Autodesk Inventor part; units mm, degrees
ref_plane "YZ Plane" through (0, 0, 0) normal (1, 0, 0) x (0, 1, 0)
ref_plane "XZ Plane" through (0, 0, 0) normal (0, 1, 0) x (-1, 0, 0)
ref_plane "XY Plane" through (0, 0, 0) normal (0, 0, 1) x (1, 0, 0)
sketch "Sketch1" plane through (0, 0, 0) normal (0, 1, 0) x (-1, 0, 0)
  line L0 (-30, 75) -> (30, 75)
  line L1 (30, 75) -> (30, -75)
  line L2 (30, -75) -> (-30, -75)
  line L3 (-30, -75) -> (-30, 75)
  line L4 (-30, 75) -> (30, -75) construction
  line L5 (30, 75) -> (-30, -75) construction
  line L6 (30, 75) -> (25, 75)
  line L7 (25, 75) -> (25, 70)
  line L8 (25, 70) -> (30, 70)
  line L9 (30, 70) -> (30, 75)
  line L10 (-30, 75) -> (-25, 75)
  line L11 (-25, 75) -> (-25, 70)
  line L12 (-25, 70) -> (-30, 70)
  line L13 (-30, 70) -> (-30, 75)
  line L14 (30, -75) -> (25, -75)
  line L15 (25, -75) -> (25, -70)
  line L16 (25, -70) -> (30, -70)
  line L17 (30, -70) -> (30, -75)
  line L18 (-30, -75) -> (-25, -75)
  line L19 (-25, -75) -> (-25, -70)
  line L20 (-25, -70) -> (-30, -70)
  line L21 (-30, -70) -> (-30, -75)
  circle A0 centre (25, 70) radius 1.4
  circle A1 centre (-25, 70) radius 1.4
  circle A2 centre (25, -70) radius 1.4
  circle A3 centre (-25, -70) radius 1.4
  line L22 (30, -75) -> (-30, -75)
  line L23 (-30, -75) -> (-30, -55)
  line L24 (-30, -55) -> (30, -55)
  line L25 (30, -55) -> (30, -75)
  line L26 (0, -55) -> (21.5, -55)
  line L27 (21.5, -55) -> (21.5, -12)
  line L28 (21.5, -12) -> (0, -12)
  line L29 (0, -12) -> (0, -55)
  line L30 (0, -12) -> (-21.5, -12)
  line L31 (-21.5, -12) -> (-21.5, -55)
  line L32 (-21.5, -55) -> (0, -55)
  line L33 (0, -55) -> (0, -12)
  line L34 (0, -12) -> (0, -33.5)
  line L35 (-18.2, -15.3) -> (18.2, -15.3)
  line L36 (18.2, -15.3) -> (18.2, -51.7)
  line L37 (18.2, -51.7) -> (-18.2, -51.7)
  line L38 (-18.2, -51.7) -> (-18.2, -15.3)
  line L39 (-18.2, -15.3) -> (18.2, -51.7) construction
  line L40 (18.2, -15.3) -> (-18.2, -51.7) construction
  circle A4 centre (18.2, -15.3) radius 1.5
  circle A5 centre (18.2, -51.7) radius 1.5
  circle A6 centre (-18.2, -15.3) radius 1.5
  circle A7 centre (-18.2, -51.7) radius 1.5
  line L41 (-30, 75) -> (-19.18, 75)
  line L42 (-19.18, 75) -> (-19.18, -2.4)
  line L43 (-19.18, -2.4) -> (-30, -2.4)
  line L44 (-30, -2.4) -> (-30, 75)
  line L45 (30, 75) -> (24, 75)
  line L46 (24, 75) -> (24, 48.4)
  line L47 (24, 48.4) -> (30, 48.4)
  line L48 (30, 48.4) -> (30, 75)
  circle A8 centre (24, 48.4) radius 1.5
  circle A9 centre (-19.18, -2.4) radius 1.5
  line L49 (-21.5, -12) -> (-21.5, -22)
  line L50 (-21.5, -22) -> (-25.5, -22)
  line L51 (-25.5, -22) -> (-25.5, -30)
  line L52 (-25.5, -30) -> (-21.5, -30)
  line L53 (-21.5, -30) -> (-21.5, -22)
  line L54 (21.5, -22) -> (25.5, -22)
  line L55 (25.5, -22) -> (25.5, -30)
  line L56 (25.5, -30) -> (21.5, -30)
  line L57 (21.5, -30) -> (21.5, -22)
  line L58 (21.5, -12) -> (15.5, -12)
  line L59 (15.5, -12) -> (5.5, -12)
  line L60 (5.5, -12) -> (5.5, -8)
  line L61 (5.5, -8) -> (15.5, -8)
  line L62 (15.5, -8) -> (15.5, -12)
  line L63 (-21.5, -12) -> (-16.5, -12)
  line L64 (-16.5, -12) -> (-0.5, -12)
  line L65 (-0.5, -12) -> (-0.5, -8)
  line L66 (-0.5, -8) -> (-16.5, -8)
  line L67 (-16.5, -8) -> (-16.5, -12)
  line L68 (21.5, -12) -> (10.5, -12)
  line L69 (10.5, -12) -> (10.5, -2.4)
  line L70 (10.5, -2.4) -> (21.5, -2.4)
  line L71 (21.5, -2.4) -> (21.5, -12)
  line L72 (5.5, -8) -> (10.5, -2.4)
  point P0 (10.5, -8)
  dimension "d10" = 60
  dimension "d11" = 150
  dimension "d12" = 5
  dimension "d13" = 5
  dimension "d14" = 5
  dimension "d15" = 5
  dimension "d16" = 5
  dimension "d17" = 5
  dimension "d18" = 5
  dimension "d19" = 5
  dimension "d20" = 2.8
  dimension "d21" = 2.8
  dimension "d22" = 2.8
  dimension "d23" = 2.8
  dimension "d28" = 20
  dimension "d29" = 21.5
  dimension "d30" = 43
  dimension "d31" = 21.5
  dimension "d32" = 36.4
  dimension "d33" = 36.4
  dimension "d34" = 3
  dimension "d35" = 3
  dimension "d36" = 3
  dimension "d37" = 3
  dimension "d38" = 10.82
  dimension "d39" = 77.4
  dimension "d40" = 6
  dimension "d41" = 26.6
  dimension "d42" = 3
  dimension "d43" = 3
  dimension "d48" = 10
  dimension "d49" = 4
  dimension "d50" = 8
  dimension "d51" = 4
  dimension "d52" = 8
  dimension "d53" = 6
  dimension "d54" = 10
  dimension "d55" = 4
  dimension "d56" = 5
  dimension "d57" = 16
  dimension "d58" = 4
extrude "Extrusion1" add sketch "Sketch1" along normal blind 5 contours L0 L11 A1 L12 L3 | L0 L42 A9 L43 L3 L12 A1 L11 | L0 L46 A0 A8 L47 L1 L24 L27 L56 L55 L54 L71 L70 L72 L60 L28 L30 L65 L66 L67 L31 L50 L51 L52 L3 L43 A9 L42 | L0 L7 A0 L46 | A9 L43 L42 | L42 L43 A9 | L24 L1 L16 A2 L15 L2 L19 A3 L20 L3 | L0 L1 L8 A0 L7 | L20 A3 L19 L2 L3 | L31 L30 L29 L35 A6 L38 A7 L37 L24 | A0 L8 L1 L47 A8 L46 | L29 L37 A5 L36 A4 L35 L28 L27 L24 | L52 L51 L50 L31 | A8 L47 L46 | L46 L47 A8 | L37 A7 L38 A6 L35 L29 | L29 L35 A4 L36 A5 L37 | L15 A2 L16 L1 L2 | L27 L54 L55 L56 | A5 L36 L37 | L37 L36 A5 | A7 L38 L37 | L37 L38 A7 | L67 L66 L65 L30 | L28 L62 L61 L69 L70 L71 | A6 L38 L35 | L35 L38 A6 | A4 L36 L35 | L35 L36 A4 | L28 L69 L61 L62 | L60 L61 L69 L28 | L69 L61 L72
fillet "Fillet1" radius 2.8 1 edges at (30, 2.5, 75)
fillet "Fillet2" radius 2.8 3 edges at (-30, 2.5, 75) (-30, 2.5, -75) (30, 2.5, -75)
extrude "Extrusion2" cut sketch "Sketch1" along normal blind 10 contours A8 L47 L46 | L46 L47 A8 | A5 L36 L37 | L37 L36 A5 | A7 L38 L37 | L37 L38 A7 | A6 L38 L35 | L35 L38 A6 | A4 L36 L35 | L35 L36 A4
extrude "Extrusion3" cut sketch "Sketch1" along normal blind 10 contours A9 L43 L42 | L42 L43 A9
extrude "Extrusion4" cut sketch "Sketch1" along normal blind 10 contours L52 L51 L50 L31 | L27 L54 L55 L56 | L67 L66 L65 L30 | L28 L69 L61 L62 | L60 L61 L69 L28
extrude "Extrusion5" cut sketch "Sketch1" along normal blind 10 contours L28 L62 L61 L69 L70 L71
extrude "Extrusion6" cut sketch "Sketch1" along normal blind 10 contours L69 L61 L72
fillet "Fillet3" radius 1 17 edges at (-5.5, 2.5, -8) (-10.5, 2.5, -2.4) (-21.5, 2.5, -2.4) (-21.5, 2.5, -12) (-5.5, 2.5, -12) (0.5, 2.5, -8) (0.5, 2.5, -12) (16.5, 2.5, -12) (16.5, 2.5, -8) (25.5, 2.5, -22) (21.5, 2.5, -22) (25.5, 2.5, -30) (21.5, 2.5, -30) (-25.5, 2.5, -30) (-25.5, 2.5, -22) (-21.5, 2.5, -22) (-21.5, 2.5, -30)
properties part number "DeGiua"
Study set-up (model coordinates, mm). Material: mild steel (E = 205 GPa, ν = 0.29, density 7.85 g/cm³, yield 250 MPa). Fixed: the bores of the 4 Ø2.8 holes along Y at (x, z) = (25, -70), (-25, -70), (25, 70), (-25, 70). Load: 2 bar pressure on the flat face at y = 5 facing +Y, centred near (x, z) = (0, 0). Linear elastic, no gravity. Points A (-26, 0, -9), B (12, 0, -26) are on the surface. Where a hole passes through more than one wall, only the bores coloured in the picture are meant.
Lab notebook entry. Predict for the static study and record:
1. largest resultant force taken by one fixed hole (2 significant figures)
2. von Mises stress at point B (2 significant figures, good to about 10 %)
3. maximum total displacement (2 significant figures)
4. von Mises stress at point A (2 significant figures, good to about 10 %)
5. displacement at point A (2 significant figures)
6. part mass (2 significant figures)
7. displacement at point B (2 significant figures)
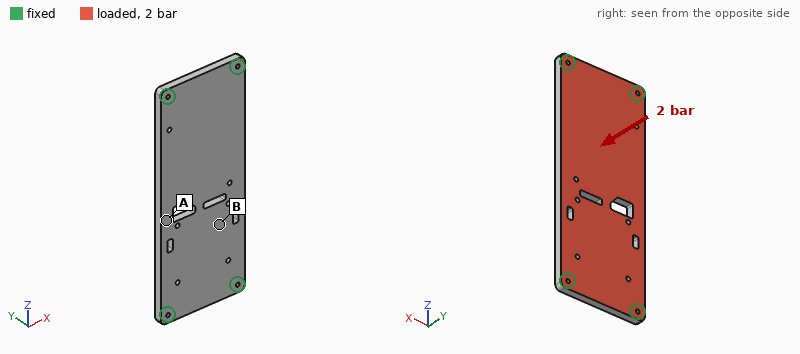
440 N
23 MPa
0.15 mm
72 MPa
0.14 mm
340 g
0.11 mm
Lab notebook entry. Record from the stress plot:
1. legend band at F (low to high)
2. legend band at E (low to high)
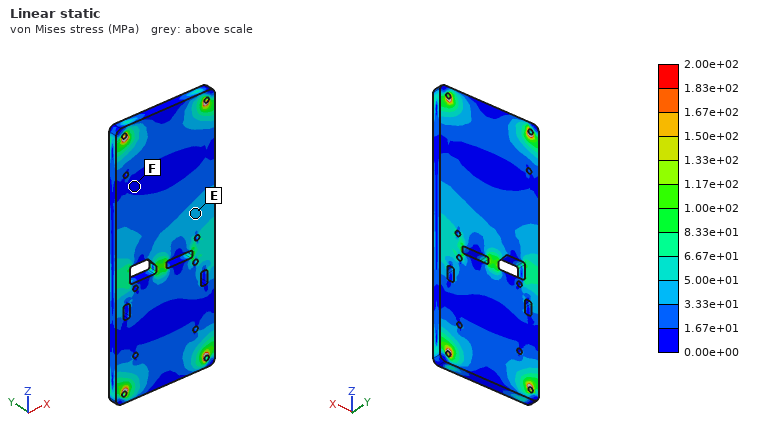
0.00e+00 to 1.67e+01 MPa
3.33e+01 to 5.00e+01 MPa
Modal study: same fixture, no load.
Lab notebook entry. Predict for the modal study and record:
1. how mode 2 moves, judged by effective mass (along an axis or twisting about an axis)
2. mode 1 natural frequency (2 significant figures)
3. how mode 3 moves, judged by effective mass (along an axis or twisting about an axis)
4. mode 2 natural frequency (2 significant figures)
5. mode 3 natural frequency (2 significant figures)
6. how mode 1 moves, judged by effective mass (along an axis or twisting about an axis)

twisting about Z
1100 Hz
twisting about X
2400 Hz
3100 Hz
along Y
